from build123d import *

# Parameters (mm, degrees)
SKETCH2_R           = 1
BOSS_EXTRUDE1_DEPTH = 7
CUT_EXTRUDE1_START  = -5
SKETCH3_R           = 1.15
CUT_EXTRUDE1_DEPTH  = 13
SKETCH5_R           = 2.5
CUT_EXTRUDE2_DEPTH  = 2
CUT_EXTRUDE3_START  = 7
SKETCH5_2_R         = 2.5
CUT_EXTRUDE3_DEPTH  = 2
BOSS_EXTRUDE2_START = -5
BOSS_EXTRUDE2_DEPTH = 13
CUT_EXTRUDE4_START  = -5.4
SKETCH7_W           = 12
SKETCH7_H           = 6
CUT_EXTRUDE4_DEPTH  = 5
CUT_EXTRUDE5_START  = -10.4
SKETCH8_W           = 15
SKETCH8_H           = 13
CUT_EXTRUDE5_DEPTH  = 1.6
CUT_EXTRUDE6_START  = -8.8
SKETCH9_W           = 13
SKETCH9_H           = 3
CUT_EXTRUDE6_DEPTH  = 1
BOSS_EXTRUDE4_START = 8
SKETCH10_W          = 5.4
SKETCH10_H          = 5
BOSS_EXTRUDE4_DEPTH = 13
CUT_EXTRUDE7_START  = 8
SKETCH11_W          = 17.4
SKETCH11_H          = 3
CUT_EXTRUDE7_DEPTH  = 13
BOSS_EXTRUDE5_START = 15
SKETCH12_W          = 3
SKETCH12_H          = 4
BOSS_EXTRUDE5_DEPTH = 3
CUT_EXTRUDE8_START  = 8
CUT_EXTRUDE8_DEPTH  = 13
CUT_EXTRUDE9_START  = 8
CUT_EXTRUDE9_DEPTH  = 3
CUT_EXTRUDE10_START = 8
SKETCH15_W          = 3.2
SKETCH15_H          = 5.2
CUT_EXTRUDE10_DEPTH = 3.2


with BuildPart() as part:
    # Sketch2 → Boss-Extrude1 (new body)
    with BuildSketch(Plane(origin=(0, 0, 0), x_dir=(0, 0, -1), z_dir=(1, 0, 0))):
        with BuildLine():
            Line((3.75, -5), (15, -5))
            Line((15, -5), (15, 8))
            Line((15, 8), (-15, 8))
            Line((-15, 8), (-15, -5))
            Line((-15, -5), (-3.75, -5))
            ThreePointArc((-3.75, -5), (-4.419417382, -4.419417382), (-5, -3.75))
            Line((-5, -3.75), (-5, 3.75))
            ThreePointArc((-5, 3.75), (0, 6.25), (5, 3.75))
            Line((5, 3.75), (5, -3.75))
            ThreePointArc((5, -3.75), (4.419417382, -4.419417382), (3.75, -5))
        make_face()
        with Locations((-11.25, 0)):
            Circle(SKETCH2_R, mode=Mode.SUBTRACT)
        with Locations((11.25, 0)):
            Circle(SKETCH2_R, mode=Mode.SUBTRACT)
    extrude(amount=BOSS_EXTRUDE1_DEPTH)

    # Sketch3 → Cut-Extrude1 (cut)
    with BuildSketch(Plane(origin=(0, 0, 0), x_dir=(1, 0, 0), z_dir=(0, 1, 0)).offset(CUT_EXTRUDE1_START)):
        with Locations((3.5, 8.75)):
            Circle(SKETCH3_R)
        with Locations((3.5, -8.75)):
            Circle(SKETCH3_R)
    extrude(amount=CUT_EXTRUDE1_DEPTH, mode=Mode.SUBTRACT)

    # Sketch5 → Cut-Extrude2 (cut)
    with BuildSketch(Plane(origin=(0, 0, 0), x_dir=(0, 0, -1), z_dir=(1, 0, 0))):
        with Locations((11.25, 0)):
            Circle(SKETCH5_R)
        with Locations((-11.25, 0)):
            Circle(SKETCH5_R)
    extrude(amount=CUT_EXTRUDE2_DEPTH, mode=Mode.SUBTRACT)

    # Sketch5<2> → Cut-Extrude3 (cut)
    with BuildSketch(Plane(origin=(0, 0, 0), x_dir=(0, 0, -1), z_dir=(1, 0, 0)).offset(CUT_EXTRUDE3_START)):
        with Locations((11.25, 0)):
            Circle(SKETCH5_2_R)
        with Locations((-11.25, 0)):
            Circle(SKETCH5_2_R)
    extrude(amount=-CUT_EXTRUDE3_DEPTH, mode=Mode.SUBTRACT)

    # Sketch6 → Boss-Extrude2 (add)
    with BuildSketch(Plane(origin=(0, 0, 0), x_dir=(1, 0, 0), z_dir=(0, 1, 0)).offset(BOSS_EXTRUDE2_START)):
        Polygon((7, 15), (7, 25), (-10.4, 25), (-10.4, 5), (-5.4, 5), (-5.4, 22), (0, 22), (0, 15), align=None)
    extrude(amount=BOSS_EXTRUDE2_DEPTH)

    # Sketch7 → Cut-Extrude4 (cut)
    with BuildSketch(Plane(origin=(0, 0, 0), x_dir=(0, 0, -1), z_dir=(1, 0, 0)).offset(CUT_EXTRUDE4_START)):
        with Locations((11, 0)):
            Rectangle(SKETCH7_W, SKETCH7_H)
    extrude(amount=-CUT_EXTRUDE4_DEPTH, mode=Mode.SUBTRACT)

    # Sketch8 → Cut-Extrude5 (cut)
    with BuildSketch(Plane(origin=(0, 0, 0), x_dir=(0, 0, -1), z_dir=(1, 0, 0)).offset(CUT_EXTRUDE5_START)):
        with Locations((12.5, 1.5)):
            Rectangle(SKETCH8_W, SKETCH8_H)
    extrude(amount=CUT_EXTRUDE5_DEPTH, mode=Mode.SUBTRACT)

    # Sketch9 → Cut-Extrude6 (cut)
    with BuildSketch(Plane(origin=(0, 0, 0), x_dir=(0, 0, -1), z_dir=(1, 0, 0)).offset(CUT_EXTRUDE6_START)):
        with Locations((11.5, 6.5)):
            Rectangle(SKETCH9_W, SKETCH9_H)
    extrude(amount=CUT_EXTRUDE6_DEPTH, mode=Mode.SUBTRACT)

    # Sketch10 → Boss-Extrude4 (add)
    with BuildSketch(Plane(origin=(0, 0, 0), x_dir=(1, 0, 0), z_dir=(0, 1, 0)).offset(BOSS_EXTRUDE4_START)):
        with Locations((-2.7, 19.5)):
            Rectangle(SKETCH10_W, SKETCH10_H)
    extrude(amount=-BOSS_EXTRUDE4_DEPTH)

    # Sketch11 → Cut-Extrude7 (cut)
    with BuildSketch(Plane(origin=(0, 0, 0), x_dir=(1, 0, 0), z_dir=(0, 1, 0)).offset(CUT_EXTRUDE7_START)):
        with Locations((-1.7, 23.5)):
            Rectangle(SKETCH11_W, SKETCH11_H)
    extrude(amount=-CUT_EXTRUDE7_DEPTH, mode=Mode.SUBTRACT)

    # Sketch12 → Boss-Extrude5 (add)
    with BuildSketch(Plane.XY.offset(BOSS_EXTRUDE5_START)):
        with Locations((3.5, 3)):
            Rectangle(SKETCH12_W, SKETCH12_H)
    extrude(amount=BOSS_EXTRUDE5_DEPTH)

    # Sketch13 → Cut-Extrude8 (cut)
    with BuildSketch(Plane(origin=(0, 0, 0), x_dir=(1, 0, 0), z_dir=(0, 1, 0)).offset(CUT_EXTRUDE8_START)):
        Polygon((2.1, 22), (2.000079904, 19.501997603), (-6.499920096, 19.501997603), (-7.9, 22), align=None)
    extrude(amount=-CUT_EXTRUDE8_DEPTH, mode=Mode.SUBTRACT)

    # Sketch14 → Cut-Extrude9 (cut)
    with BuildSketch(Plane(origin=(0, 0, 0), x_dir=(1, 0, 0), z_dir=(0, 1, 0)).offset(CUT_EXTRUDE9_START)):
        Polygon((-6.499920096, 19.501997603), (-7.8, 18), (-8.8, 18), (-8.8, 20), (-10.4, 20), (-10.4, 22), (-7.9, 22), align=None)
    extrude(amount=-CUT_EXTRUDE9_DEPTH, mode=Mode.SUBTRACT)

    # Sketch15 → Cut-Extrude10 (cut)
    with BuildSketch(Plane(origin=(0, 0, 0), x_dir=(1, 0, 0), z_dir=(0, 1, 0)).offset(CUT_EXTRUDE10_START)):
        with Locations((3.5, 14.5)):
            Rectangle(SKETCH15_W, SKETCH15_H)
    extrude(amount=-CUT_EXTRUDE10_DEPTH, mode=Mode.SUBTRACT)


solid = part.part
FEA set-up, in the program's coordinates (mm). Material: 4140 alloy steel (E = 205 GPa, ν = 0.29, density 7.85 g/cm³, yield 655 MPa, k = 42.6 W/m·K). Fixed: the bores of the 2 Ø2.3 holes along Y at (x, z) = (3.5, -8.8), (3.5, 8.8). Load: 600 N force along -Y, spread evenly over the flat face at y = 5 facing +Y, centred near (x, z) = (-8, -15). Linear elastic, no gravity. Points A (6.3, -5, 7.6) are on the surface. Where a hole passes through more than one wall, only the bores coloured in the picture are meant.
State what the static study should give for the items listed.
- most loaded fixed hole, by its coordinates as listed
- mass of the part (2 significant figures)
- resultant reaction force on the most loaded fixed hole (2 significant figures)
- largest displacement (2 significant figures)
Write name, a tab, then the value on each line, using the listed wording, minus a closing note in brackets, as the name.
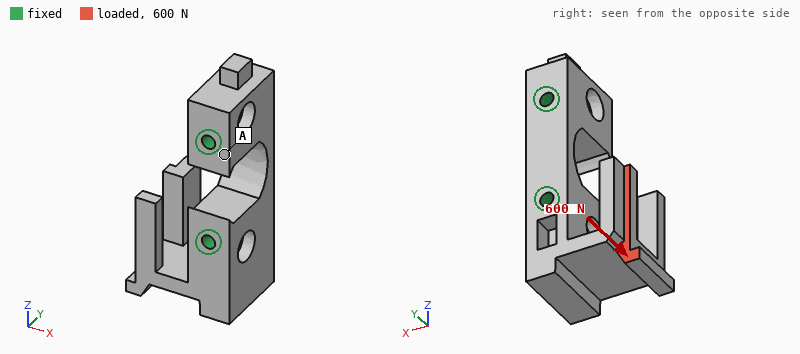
most loaded fixed hole, by its coordinates as listed	(3.5, -8.8)
mass of the part	23 g
resultant reaction force on the most loaded fixed hole	600 N
largest displacement	83 µm
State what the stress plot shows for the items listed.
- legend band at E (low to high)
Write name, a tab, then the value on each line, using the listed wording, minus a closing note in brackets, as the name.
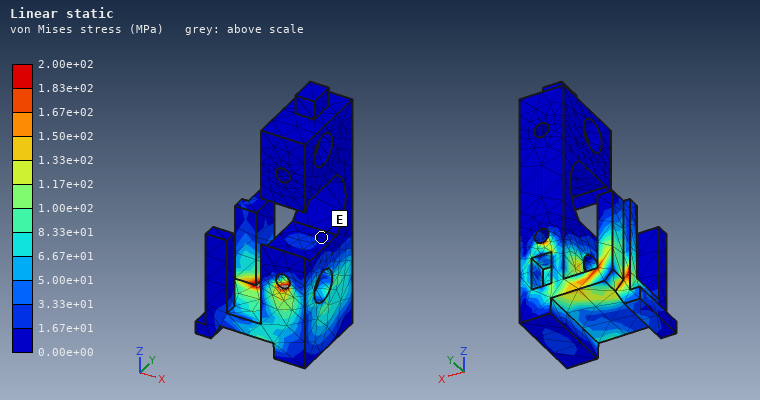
legend band at E	0.00e+00 to 1.67e+01 MPa
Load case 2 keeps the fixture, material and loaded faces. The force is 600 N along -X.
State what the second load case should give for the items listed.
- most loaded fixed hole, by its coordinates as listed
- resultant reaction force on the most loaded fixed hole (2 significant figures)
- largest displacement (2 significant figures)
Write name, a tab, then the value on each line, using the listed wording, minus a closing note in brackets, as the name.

most loaded fixed hole, by its coordinates as listed	(3.5, -8.8)
resultant reaction force on the most loaded fixed hole	640 N
largest displacement	0.11 mm
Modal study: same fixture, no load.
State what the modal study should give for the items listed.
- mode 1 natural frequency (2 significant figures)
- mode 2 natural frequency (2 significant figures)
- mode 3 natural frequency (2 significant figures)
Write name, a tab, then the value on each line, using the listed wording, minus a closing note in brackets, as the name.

mode 1 natural frequency	6500 Hz
mode 2 natural frequency	8100 Hz
mode 3 natural frequency	11 kHz
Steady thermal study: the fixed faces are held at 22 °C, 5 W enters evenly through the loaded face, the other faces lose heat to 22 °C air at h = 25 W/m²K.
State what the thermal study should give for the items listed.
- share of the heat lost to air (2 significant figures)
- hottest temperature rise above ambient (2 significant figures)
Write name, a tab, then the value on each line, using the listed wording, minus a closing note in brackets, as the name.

share of the heat lost to air	17 %
hottest temperature rise above ambient	73 K
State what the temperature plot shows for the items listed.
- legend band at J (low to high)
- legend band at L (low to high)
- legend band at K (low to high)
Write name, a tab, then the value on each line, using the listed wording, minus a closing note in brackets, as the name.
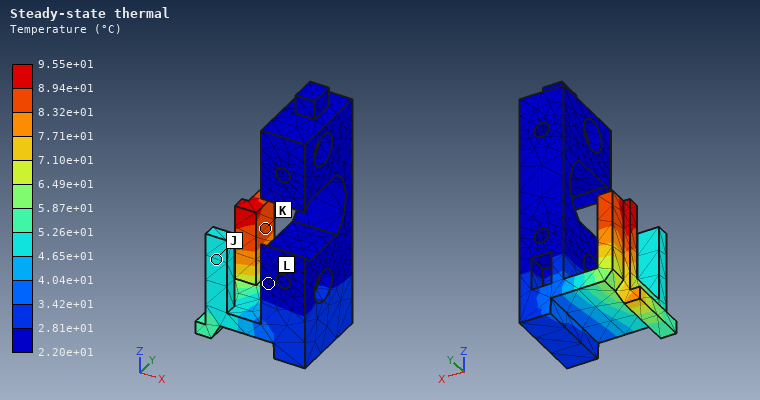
legend band at J	4.65e+01 to 5.26e+01 °C
legend band at L	2.20e+01 to 2.81e+01 °C
legend band at K	8.32e+01 to 8.94e+01 °C
